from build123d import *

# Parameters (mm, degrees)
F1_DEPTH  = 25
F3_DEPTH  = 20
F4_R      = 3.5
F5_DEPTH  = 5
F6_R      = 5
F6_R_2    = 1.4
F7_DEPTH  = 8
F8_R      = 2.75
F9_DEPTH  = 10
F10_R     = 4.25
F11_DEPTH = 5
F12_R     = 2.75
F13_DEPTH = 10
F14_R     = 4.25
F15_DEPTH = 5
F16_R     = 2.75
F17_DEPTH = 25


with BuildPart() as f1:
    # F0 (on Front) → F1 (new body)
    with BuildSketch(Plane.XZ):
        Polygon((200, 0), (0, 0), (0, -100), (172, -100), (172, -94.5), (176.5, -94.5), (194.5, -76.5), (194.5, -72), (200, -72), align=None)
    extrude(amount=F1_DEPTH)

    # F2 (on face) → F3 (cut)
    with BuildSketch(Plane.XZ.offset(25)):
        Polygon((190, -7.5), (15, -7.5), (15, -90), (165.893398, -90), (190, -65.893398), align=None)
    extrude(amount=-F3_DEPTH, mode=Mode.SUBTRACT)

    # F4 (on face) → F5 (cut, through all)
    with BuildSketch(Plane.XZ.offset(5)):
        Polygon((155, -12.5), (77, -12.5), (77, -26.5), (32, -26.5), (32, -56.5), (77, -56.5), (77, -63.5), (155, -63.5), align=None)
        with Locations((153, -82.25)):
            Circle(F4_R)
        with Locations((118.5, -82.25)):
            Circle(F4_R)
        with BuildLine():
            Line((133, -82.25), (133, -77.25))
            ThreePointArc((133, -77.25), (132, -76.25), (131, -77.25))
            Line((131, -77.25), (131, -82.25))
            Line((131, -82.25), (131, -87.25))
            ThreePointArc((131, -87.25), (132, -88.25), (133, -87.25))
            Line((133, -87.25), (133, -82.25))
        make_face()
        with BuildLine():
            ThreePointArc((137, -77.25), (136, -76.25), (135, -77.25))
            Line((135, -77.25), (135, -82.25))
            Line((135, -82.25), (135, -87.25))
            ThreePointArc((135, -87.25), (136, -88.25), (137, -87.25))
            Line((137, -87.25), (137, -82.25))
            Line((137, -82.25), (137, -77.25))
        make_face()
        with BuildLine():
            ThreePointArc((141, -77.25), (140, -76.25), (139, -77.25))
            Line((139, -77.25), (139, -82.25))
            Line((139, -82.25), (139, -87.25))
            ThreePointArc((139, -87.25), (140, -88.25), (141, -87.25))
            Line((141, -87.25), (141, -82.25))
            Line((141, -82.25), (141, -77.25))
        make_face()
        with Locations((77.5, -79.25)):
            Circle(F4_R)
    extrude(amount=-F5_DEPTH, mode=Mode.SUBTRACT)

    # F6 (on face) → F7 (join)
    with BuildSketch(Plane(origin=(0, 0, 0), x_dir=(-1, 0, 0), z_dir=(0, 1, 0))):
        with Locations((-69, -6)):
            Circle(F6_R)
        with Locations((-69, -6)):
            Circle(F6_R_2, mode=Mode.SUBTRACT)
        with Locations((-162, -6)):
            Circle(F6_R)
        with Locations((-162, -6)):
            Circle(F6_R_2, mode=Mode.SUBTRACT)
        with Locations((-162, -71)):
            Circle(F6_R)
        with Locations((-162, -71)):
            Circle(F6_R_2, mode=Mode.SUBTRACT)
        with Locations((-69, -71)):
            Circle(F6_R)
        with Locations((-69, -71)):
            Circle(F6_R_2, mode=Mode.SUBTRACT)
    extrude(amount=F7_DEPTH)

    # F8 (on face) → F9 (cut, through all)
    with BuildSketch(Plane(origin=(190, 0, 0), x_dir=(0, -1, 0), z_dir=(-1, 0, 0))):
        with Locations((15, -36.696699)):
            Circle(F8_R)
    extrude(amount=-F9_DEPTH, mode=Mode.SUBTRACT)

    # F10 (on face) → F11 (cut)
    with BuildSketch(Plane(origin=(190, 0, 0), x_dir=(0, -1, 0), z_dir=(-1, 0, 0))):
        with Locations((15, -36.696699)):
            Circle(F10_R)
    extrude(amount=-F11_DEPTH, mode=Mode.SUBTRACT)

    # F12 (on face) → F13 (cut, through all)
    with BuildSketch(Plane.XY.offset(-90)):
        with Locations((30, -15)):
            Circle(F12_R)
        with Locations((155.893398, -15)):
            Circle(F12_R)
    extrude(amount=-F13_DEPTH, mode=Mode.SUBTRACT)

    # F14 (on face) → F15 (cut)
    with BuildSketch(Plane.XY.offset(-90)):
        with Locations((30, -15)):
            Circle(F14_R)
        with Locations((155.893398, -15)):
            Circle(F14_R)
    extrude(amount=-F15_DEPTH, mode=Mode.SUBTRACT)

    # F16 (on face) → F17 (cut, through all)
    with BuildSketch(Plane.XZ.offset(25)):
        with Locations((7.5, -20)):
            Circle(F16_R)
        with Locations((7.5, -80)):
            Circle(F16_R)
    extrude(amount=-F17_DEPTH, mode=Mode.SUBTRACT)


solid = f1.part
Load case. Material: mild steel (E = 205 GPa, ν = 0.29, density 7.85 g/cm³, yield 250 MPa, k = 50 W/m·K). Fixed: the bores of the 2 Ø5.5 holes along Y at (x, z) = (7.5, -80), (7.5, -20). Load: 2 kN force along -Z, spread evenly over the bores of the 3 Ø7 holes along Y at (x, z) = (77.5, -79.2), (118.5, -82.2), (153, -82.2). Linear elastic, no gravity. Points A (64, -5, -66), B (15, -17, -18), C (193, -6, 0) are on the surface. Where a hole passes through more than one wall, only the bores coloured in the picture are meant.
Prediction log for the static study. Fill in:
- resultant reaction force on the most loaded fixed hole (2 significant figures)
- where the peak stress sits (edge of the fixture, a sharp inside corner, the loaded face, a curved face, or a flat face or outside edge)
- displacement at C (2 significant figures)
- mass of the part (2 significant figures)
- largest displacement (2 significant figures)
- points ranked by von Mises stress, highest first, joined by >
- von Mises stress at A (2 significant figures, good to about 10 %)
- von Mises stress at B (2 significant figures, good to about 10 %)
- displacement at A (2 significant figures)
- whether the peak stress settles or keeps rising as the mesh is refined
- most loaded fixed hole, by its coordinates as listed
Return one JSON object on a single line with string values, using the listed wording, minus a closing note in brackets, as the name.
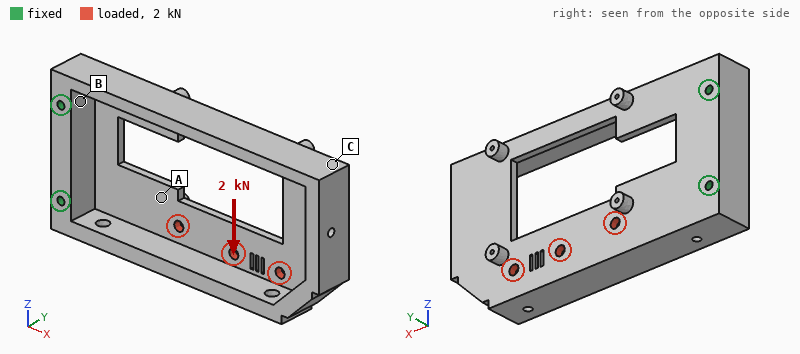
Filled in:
{"resultant reaction force on the most loaded fixed hole": "3.4 kN", "where the peak stress sits": "edge of the fixture", "displacement at C": "0.098 mm", "mass of the part": "1.4 kg", "largest displacement": "0.12 mm", "points ranked by von Mises stress, highest first, joined by >": "A > B > C", "von Mises stress at A": "21 MPa", "von Mises stress at B": "13 MPa", "displacement at A": "0.029 mm", "whether the peak stress settles or keeps rising as the mesh is refined": "keeps rising", "most loaded fixed hole, by its coordinates as listed": "(7.5, -20)"}
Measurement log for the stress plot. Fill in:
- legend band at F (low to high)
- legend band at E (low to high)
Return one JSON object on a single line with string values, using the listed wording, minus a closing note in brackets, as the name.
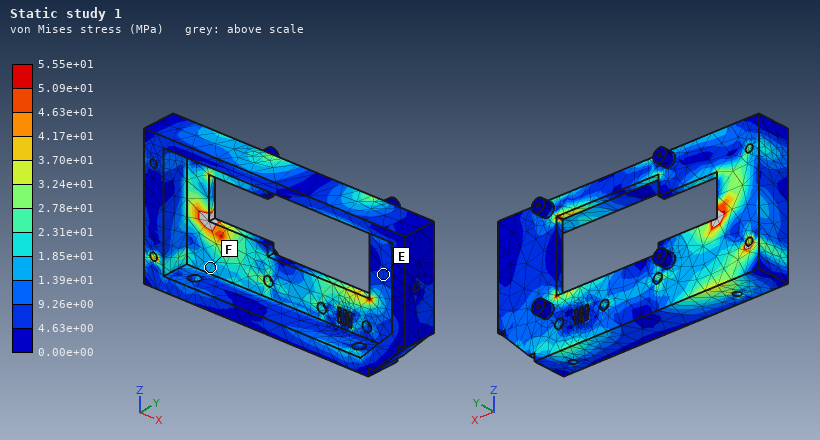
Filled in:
{"legend band at F": "1.39e+01 to 1.85e+01 MPa", "legend band at E": "4.63e+00 to 9.26e+00 MPa"}
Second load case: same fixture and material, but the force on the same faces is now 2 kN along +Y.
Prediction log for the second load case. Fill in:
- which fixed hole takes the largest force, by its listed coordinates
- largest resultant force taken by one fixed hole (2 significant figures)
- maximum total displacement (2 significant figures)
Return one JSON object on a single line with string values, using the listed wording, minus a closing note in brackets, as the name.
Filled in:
{"which fixed hole takes the largest force, by its listed coordinates": "(7.5, -80)", "largest resultant force taken by one fixed hole": "1.8 kN", "maximum total displacement": "0.42 mm"}
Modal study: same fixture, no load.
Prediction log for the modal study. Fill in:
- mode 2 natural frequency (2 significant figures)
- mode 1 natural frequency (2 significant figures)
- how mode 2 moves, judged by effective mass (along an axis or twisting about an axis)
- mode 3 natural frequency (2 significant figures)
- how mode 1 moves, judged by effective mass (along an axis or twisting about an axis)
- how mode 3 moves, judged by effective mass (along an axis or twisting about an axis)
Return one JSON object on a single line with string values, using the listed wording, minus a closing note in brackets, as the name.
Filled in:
{"mode 2 natural frequency": "620 Hz", "mode 1 natural frequency": "390 Hz", "how mode 2 moves, judged by effective mass": "along Z", "mode 3 natural frequency": "1000 Hz", "how mode 1 moves, judged by effective mass": "along Y", "how mode 3 moves, judged by effective mass": "along Z"}
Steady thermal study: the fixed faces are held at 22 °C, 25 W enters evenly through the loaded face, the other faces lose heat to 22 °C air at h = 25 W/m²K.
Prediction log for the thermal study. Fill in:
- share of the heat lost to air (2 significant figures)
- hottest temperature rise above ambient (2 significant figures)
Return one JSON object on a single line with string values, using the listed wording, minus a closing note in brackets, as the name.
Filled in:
{"share of the heat lost to air": "73 %", "hottest temperature rise above ambient": "41 K"}
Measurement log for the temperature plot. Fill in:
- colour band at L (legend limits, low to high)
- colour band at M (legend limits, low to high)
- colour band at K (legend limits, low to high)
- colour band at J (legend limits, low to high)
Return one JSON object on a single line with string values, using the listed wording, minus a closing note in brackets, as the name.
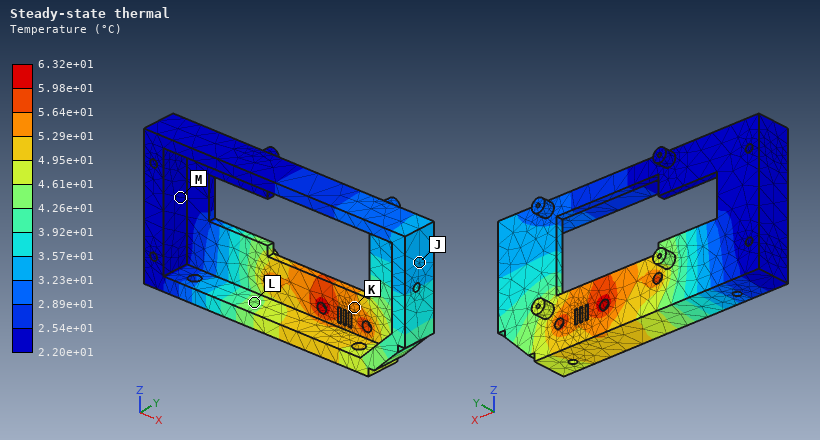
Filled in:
{"colour band at L": "4.26e+01 to 4.61e+01 °C", "colour band at M": "2.20e+01 to 2.54e+01 °C", "colour band at K": "5.29e+01 to 5.64e+01 °C", "colour band at J": "3.23e+01 to 3.57e+01 °C"}
